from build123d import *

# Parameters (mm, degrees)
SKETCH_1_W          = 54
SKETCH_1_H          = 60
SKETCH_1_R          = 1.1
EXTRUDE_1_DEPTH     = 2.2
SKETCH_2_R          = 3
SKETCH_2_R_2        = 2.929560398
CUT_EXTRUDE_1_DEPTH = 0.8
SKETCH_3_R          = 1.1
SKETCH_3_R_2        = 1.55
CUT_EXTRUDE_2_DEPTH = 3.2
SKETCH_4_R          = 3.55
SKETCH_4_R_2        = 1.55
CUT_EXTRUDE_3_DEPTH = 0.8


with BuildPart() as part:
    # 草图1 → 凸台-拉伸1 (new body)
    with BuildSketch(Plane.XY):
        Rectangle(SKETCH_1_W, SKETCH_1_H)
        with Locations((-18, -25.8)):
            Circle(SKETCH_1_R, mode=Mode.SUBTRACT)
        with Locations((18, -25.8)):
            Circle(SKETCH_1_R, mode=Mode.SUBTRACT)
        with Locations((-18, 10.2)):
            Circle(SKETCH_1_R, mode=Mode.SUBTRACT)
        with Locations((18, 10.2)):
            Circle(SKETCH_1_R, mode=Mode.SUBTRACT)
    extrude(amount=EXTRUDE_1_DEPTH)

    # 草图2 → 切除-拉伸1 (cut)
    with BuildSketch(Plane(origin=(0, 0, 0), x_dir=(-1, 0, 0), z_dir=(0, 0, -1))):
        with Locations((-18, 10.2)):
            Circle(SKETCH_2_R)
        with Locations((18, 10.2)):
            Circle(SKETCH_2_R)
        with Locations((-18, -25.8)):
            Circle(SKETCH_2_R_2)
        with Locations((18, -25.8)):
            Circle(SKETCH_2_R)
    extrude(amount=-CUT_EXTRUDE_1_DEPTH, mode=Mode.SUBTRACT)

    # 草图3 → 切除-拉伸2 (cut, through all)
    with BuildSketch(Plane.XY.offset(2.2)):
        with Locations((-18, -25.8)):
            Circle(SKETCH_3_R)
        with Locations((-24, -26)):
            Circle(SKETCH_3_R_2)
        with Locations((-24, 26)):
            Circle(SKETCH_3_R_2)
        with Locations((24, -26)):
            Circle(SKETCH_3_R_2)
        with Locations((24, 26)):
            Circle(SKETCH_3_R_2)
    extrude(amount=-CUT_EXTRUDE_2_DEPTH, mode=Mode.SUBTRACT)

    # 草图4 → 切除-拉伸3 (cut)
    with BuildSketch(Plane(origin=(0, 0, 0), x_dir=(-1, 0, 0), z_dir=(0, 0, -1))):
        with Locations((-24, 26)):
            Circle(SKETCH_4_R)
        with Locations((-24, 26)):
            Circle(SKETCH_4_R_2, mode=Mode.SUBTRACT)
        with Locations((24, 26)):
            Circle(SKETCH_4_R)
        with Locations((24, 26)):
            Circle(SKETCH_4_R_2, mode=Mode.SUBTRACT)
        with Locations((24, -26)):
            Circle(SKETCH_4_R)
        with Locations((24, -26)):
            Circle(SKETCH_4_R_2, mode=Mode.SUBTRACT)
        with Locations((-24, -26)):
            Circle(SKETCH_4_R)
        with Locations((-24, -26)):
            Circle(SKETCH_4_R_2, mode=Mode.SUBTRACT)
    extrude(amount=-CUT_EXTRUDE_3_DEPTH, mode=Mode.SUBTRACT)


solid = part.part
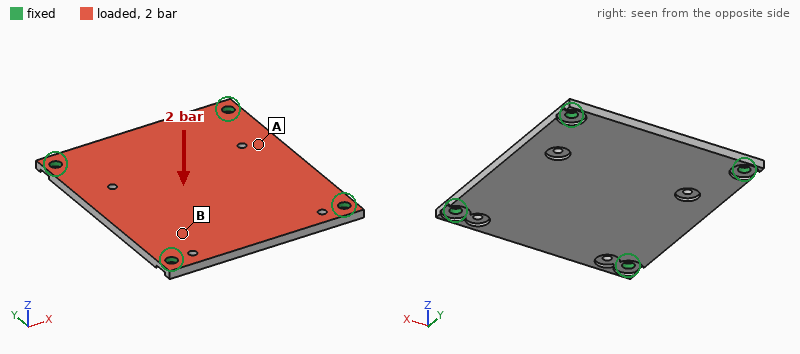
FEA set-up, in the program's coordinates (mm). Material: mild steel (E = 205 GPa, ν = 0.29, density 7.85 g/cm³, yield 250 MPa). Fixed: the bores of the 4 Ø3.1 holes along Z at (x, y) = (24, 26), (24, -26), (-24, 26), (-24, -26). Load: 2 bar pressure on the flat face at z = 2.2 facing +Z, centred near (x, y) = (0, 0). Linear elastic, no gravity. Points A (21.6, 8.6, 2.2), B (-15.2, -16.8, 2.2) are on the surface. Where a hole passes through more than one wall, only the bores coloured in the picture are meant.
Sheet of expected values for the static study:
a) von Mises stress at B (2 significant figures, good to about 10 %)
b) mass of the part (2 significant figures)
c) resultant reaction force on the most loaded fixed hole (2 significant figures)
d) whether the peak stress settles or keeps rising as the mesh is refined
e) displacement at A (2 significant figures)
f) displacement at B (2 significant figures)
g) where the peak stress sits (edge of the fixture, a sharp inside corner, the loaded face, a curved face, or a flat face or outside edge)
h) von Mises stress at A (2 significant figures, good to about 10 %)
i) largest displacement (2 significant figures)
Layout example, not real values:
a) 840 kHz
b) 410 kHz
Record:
a) 15 MPa
b) 54 g
c) 310 N
d) keeps rising
e) 41 µm
f) 33 µm
g) edge of the fixture
h) 38 MPa
i) 66 µm
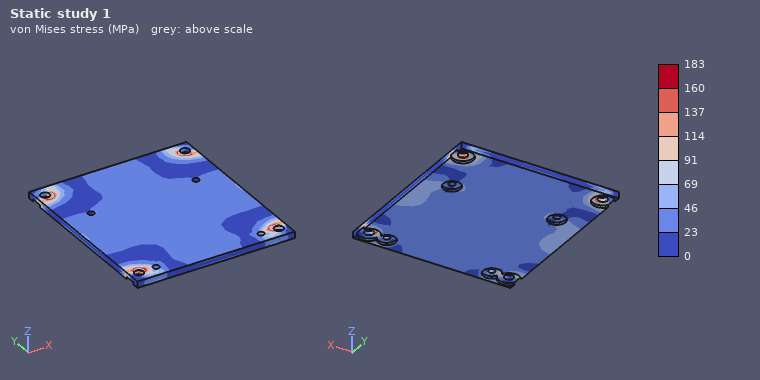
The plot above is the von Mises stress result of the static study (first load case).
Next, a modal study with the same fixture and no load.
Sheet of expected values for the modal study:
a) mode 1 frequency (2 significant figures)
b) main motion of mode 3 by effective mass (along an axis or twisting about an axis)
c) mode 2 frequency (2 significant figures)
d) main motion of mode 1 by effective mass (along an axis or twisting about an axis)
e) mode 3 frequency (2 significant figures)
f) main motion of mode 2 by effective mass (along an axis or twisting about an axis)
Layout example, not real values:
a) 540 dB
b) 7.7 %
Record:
a) 2500 Hz
b) twisting about X
c) 4300 Hz
d) along Z
e) 4700 Hz
f) twisting about Y
